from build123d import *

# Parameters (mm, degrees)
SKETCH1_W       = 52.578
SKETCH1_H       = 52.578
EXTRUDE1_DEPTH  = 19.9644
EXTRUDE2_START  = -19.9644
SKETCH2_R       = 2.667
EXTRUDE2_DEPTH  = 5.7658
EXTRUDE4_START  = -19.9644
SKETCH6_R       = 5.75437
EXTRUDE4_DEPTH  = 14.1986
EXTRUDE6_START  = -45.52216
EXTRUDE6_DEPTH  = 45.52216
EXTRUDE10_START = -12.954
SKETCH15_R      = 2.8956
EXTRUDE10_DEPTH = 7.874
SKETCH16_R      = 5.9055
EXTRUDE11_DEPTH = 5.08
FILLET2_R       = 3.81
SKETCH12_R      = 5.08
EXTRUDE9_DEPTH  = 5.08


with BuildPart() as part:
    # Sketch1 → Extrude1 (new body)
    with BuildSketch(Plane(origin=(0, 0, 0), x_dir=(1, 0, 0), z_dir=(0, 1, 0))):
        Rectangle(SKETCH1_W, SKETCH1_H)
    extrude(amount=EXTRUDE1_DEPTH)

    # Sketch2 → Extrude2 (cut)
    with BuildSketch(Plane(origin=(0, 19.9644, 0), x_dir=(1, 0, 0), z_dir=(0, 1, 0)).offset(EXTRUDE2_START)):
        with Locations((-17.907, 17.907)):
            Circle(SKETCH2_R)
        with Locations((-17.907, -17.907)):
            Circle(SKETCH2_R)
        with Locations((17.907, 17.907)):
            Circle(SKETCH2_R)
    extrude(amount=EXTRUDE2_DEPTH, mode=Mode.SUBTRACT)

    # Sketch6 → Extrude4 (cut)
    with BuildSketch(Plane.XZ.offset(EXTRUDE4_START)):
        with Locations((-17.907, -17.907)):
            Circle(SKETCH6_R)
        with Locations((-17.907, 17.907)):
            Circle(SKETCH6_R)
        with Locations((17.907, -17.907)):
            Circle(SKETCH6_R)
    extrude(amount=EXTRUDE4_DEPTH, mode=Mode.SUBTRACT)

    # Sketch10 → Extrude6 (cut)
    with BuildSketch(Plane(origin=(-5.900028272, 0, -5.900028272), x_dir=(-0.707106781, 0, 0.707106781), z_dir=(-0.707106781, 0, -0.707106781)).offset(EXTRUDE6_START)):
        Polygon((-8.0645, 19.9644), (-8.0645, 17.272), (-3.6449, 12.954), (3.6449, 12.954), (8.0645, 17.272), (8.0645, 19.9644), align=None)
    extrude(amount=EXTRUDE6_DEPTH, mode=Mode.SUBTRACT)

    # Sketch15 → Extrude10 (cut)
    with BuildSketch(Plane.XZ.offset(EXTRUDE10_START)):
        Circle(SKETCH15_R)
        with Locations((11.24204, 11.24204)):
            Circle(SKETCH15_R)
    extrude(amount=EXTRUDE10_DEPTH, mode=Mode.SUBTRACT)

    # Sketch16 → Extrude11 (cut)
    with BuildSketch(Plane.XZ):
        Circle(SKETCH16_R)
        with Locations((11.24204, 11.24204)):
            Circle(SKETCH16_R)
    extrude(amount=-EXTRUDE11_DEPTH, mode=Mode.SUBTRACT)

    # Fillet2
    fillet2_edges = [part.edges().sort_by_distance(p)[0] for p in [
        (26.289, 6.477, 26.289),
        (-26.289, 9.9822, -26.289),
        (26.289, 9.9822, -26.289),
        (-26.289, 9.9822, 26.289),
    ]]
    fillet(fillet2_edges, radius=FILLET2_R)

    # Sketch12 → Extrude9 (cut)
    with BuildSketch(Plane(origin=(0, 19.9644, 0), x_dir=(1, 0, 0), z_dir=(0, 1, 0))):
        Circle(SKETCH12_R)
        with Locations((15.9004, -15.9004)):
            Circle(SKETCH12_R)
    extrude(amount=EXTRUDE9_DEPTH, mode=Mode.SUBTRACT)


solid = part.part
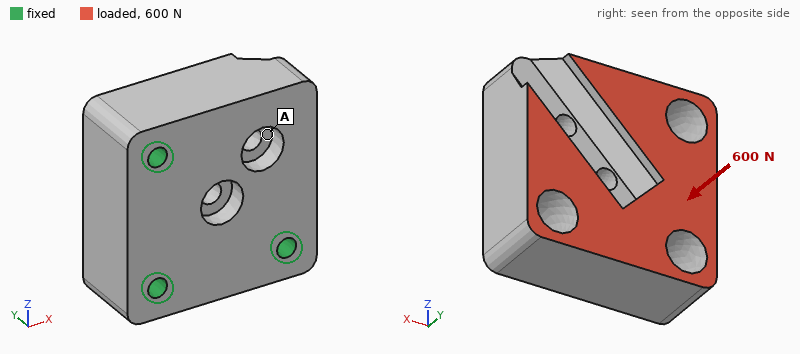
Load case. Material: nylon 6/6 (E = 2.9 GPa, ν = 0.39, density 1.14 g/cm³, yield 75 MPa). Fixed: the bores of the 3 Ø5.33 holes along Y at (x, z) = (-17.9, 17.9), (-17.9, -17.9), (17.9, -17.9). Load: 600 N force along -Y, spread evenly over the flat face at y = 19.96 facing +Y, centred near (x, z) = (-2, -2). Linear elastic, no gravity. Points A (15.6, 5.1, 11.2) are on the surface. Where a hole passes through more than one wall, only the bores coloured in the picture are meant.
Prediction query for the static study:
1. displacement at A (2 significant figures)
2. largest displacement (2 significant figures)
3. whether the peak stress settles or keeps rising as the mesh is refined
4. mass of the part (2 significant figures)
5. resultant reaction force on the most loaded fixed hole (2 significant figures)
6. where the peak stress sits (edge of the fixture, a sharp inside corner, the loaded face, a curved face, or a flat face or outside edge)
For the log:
42 µm
64 µm
keeps rising
51 g
270 N
edge of the fixture
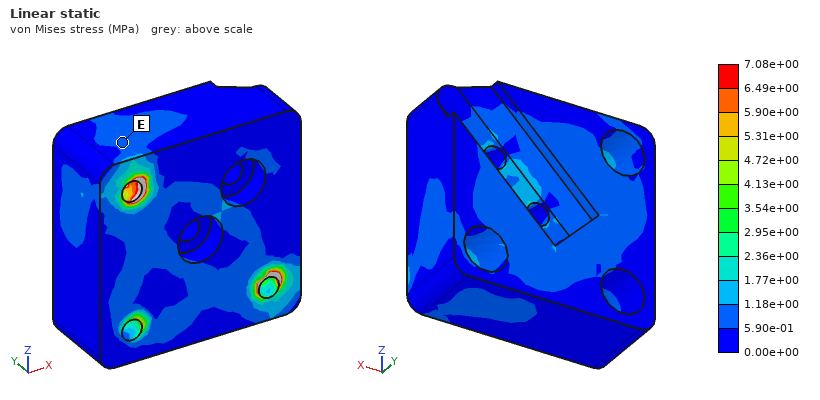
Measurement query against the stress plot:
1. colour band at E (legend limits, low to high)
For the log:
5.90e-01 to 1.18e+00 MPa
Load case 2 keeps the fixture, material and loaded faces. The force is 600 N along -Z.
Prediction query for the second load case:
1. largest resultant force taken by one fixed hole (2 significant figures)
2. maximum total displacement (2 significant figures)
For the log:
360 N
81 µm
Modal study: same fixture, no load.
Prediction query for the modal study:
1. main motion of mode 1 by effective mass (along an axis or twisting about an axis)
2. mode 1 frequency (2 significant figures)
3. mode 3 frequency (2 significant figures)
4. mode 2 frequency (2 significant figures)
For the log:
along Y
2300 Hz
5600 Hz
5100 Hz
